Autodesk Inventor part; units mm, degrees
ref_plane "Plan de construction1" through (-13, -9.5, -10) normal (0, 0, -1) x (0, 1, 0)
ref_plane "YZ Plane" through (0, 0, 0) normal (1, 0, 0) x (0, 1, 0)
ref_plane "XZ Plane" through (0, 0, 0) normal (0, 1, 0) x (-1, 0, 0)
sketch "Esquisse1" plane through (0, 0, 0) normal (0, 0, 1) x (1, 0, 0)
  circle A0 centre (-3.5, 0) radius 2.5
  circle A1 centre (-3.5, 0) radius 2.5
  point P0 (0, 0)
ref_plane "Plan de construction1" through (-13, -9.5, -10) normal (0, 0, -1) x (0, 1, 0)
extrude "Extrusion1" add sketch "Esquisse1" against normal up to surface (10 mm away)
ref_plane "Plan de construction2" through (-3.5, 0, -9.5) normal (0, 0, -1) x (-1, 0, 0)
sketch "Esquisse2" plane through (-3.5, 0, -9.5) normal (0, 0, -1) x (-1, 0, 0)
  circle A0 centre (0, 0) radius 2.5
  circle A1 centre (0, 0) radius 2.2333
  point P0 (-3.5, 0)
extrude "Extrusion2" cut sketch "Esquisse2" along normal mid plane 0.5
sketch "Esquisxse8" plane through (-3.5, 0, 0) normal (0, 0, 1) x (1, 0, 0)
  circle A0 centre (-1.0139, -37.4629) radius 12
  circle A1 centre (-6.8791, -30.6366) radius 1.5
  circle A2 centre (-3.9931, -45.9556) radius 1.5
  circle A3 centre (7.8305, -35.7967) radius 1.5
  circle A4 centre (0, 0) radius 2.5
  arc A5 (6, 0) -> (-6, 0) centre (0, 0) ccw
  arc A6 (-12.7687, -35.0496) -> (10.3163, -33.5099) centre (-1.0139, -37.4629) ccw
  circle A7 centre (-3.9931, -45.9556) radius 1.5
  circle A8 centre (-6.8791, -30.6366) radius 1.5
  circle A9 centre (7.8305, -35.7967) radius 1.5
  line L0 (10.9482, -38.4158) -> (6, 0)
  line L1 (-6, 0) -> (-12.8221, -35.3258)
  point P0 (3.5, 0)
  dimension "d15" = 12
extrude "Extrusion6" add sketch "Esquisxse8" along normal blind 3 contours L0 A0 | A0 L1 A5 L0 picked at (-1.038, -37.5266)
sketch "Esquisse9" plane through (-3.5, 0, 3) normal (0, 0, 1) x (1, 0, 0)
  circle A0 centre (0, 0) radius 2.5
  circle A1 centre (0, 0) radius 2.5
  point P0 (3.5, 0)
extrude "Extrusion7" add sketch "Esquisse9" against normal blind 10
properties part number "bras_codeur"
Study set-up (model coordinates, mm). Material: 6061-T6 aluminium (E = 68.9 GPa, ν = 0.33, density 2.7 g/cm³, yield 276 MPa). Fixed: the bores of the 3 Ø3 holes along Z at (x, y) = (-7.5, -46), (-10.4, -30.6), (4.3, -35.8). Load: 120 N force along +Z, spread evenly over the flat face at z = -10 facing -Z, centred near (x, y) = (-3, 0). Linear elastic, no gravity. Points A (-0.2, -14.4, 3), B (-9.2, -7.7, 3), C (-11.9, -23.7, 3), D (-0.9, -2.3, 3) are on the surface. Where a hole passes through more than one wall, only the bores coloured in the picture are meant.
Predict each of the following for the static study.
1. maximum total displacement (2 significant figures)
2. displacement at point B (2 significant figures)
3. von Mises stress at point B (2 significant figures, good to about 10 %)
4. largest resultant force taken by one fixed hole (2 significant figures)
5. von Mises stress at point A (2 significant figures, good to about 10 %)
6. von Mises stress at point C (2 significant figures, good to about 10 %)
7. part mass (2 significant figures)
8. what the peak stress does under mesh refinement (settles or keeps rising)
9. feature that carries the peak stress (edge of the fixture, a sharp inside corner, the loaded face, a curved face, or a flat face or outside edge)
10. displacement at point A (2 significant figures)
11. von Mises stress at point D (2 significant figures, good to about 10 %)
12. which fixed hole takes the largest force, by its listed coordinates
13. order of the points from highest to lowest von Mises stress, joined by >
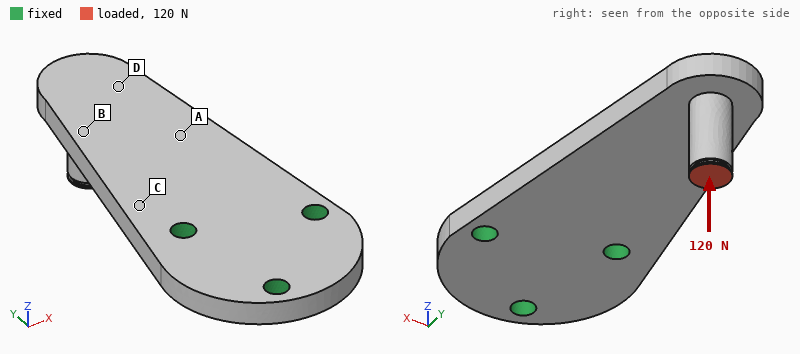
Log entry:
0.56 mm
0.26 mm
46 MPa
180 N
69 MPa
110 MPa
8.1 g
keeps rising
edge of the fixture
0.16 mm
19 MPa
(-10.4, -30.6)
C > A > B > D
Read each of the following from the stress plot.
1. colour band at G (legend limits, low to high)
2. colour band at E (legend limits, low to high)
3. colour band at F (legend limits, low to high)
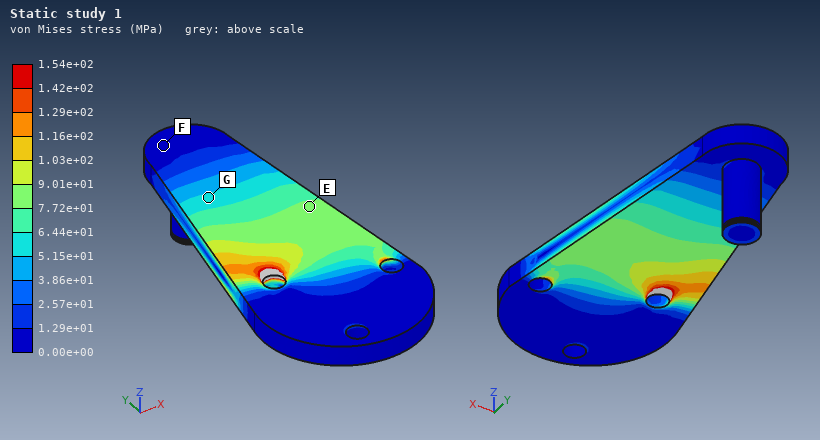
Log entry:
5.15e+01 to 6.44e+01 MPa
7.72e+01 to 9.01e+01 MPa
0.00e+00 to 1.29e+01 MPa
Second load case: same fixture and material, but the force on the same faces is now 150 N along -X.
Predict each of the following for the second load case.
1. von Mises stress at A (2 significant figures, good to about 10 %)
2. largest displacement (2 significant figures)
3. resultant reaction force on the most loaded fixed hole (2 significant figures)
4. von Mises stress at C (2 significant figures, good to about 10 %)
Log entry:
60 MPa
0.22 mm
320 N
47 MPa
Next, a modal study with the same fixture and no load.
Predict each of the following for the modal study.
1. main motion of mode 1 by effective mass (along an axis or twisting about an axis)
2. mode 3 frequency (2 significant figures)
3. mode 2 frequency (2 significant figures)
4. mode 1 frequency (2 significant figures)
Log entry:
along Z
9300 Hz
7300 Hz
1900 Hz
